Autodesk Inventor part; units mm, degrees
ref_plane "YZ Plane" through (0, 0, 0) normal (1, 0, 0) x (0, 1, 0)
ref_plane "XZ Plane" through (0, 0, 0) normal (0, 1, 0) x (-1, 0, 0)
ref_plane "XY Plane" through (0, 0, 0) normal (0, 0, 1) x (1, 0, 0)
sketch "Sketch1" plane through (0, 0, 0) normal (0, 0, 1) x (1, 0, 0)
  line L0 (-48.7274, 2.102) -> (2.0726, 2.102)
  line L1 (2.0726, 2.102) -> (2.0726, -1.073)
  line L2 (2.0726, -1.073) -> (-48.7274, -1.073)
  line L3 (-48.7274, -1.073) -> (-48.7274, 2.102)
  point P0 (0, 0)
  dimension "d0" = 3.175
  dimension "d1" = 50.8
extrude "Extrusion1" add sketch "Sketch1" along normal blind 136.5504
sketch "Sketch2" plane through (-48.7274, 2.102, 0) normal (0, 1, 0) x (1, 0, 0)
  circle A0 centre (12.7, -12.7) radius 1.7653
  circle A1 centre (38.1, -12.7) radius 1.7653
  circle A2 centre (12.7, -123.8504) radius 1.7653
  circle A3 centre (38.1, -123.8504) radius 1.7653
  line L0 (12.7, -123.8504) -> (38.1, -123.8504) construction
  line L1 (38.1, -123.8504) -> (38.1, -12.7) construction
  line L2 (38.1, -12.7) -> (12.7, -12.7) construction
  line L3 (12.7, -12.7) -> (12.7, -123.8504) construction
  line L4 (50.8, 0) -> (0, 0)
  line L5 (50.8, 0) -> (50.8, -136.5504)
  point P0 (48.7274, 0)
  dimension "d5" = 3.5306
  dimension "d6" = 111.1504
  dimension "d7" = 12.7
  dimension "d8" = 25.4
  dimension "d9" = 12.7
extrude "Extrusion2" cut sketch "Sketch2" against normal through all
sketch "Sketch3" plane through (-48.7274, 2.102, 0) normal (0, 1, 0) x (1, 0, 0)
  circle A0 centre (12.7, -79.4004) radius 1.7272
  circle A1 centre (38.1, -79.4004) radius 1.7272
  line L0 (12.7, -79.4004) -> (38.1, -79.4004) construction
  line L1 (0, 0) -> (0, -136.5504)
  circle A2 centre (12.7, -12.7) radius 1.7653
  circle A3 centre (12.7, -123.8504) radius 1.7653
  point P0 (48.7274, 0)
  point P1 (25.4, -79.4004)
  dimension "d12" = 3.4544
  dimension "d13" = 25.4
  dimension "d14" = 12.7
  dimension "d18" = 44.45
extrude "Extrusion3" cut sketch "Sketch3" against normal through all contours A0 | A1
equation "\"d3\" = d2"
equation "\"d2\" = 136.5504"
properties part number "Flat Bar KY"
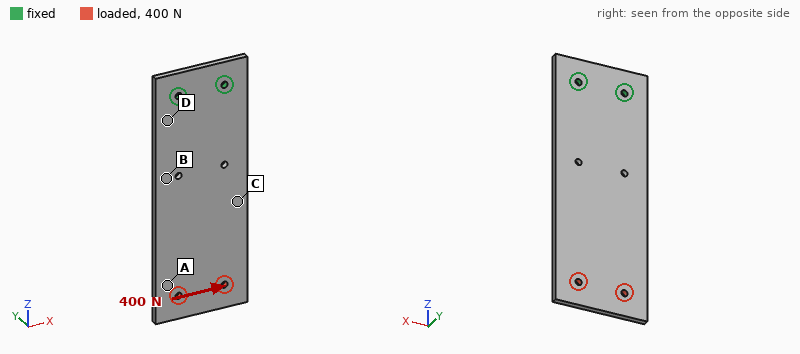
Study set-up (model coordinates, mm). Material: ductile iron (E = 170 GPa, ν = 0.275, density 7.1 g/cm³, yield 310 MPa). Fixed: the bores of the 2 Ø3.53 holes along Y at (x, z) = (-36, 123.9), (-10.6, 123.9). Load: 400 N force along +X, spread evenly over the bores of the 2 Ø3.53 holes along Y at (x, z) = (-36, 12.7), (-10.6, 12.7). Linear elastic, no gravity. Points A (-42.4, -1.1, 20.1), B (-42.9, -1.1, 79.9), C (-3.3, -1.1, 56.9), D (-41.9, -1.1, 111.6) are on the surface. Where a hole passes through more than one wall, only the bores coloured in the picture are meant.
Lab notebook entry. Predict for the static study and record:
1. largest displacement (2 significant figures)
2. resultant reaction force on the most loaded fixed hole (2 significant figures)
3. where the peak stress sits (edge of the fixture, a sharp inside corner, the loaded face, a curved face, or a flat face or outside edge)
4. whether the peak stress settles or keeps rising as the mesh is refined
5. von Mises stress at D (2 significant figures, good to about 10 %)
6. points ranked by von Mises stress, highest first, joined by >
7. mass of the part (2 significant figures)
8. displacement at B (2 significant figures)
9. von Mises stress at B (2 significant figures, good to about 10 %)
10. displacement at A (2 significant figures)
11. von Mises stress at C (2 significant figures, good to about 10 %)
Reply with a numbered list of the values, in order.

1. 56 µm
2. 1.7 kN
3. edge of the fixture
4. keeps rising
5. 22 MPa
6. D > B > C > A
7. 160 g
8. 15 µm
9. 16 MPa
10. 45 µm
11. 11 MPa
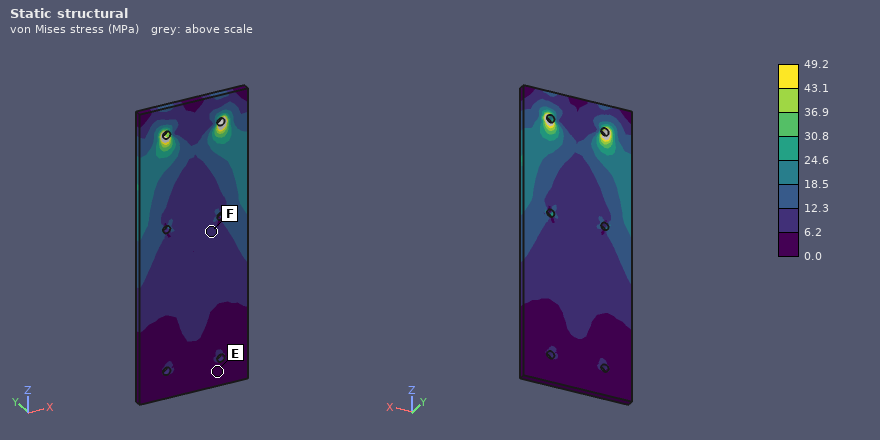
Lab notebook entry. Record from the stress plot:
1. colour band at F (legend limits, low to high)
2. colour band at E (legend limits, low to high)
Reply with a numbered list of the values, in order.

1. 6.2 to 12.3 MPa
2. 0.0 to 6.2 MPa
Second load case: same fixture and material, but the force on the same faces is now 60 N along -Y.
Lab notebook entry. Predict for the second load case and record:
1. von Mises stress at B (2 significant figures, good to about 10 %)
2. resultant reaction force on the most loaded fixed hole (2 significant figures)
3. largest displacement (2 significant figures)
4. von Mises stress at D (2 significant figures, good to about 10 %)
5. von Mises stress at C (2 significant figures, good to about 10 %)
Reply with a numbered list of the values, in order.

1. 52 MPa
2. 30 N
3. 1.4 mm
4. 67 MPa
5. 31 MPa
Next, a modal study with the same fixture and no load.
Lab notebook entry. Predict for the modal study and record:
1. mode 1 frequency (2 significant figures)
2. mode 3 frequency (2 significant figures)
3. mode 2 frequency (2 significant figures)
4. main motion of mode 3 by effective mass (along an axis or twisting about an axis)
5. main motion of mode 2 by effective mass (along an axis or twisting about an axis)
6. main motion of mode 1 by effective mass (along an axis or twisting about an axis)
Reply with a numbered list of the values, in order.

1. 160 Hz
2. 1000 Hz
3. 830 Hz
4. along Y
5. twisting about Z
6. along Y
